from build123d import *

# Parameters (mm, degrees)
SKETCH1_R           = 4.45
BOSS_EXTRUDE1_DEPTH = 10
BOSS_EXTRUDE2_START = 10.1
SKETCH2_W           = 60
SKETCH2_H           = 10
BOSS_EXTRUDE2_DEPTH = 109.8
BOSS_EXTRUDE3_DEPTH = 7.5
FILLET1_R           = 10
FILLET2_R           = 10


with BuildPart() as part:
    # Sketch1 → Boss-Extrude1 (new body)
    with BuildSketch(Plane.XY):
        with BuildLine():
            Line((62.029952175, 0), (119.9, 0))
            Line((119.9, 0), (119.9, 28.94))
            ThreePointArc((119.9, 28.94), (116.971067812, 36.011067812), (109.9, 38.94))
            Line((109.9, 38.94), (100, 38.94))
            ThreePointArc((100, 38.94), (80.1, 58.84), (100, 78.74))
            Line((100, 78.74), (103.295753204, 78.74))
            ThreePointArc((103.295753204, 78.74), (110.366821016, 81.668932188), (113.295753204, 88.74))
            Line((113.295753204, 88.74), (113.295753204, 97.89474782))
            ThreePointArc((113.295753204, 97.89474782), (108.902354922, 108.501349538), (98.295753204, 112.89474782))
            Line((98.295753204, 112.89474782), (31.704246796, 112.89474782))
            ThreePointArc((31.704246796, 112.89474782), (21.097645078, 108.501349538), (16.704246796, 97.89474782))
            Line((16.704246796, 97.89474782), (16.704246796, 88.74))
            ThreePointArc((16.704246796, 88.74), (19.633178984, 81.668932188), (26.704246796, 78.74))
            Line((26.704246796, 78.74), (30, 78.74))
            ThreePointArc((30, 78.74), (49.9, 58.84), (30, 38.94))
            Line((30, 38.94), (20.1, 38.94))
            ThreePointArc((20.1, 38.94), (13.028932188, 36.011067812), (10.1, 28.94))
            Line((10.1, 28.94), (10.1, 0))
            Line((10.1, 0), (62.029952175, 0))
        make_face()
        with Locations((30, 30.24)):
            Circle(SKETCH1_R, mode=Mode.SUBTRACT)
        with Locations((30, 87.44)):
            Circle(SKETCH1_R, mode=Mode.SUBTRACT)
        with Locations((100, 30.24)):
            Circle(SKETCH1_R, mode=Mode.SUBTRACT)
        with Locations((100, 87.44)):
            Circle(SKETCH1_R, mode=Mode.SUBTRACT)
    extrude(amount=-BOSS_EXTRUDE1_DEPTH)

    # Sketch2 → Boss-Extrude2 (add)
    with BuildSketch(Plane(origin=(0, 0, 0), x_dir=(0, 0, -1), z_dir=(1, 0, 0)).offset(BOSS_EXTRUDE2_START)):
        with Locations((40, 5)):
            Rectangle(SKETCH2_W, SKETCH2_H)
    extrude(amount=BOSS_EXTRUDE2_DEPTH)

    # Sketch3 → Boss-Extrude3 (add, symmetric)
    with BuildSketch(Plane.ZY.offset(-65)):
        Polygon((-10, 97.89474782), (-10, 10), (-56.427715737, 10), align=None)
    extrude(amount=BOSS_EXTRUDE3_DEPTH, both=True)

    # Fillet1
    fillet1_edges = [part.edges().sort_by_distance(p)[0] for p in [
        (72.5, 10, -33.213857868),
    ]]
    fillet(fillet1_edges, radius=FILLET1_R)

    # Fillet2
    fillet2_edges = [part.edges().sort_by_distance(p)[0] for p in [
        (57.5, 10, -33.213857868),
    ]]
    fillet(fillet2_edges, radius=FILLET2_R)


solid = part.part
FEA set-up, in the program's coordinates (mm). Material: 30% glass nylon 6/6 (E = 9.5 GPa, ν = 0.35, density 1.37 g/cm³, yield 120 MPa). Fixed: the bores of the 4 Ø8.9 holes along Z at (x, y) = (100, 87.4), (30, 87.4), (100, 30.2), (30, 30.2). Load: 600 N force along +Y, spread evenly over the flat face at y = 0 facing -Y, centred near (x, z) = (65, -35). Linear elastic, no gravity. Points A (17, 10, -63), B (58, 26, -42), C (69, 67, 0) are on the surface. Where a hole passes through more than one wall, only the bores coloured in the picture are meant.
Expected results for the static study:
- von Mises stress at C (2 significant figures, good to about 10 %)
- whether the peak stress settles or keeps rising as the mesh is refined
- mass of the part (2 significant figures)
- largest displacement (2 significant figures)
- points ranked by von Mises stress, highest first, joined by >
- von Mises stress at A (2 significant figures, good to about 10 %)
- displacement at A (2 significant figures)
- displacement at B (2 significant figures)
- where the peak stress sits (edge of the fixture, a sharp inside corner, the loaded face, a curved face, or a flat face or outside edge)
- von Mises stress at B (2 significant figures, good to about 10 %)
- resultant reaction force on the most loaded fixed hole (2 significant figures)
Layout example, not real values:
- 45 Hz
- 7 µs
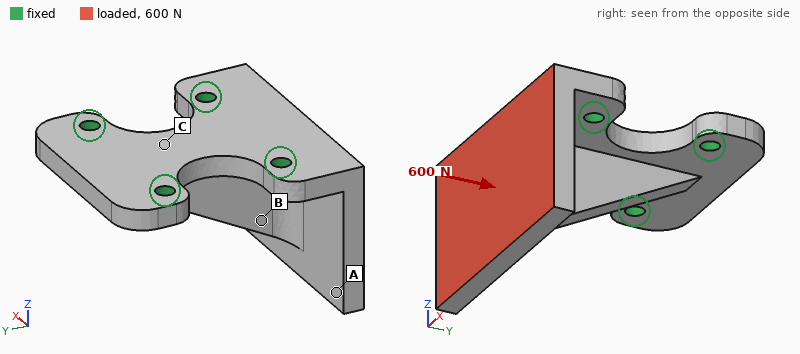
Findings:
- 0.99 MPa
- keeps rising
- 250 g
- 0.10 mm
- B > C > A
- 0.46 MPa
- 0.084 mm
- 0.029 mm
- edge of the fixture
- 1.5 MPa
- 210 N
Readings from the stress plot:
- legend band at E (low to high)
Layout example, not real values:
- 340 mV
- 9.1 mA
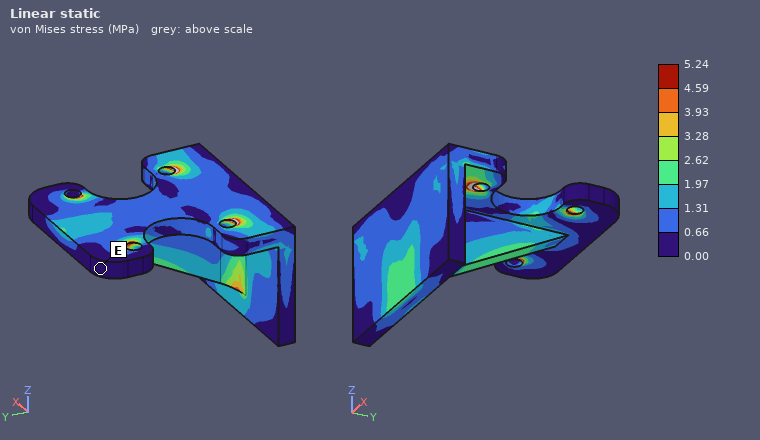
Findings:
- 0.00 to 0.66 MPa
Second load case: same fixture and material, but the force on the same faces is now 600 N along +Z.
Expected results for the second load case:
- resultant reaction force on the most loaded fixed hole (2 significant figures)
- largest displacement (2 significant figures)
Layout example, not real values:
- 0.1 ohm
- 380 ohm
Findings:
- 380 N
- 76 µm
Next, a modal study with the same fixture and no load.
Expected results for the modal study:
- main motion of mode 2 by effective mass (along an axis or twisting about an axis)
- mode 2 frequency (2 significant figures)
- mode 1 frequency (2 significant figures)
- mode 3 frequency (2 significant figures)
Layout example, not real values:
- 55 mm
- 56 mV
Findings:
- along X
- 1600 Hz
- 1400 Hz
- 2000 Hz
